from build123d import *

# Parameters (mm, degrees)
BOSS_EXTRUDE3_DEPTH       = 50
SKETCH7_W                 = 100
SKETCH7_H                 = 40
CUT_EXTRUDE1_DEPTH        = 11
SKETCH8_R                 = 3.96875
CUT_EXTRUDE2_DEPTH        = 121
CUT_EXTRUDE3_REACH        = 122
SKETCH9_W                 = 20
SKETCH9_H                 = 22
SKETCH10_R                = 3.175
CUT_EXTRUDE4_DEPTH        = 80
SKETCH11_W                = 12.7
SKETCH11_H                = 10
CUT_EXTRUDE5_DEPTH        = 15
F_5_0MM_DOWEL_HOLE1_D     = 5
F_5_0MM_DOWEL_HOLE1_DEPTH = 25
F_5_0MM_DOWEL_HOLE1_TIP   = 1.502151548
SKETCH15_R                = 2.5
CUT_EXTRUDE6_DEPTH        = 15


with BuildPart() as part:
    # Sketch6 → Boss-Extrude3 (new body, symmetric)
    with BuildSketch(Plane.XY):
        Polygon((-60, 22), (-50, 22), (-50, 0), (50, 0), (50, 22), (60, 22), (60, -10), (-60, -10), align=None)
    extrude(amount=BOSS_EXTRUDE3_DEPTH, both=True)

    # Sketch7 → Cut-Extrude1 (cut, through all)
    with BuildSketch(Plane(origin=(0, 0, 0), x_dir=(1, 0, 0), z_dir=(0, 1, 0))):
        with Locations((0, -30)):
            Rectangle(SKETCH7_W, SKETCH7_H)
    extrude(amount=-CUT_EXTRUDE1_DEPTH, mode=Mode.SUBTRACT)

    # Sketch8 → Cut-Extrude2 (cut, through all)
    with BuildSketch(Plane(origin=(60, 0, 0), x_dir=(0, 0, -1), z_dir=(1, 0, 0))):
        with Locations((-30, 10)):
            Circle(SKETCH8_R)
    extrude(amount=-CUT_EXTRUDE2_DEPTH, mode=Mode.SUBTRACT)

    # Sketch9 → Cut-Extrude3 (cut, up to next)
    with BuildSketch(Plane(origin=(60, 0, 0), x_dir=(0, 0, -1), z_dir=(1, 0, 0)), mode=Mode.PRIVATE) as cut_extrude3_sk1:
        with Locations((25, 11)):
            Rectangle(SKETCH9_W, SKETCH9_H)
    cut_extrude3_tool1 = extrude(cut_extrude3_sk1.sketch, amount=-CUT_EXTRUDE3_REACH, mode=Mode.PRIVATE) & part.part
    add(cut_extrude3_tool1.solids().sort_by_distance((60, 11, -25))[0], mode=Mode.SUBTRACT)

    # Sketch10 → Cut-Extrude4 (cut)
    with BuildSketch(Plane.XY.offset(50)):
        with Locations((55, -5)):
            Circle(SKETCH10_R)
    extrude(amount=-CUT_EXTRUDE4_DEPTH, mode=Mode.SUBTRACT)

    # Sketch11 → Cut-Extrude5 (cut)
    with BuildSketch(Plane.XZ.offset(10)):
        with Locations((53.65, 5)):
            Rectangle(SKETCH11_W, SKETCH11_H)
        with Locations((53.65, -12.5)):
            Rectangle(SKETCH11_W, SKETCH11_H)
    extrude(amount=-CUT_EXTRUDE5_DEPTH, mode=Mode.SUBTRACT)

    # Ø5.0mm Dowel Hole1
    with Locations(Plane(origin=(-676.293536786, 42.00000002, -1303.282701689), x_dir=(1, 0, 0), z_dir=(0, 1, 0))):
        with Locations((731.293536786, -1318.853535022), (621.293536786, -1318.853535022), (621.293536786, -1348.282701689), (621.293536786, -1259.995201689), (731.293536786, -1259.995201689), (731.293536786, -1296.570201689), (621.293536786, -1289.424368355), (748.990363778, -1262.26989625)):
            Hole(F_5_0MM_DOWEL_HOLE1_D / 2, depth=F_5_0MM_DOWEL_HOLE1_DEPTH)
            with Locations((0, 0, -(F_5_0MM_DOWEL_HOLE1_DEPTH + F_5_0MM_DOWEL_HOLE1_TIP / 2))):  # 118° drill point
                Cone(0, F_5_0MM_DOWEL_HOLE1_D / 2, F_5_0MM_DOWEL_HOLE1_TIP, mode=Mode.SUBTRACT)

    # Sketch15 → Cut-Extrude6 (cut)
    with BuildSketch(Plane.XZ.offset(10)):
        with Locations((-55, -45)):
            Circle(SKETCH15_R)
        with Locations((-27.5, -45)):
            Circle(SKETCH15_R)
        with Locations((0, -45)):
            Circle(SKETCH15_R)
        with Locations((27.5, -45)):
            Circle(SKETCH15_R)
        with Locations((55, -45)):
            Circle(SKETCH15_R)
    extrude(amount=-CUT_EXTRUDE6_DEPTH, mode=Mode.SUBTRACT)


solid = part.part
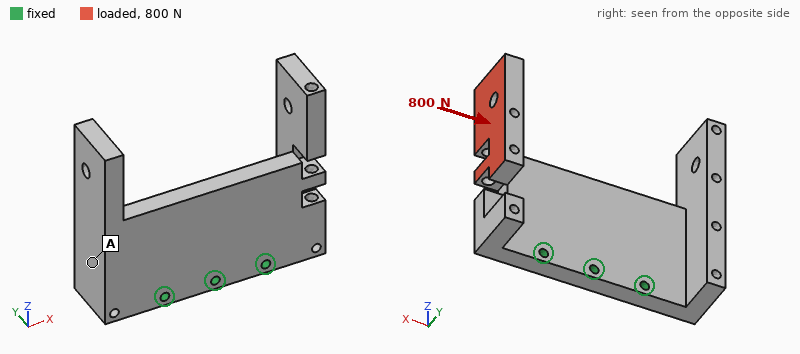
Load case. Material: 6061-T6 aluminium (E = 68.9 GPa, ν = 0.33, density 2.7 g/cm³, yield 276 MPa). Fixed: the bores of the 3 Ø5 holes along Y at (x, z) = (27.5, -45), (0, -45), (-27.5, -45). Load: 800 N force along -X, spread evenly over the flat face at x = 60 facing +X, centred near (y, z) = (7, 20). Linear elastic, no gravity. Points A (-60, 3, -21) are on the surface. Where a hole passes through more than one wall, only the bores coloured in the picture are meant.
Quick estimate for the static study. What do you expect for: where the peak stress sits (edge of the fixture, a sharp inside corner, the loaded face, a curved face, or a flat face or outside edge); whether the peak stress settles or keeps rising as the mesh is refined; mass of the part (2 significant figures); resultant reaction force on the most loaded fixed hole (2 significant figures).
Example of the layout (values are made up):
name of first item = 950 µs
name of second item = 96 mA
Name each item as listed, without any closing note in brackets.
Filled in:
where the peak stress sits = a sharp inside corner
whether the peak stress settles or keeps rising as the mesh is refined = keeps rising
mass of the part = 300 g
resultant reaction force on the most loaded fixed hole = 970 N
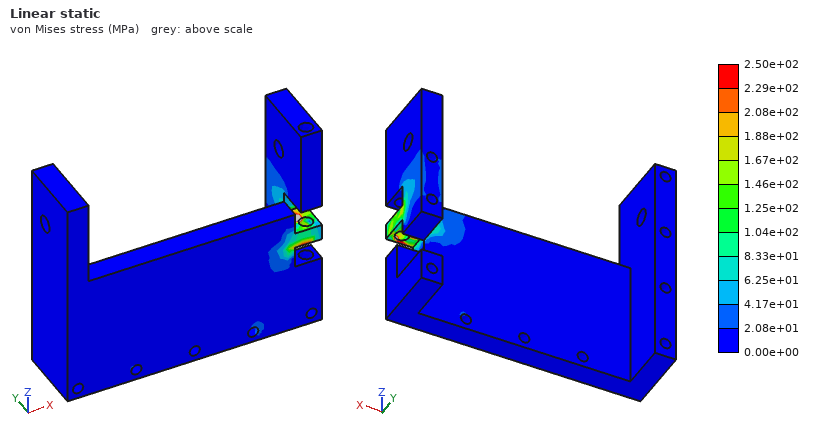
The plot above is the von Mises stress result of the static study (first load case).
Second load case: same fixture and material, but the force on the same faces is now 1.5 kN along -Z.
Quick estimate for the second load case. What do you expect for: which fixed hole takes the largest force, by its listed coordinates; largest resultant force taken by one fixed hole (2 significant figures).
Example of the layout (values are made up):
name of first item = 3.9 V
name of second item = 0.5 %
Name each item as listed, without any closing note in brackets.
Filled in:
which fixed hole takes the largest force, by its listed coordinates = (27.5, -45)
largest resultant force taken by one fixed hole = 2.3 kN
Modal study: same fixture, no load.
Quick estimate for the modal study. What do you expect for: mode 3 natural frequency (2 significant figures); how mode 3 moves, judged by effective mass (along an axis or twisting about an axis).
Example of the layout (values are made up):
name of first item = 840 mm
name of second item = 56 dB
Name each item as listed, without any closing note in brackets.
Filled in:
mode 3 natural frequency = 1000 Hz
how mode 3 moves, judged by effective mass = along Y
